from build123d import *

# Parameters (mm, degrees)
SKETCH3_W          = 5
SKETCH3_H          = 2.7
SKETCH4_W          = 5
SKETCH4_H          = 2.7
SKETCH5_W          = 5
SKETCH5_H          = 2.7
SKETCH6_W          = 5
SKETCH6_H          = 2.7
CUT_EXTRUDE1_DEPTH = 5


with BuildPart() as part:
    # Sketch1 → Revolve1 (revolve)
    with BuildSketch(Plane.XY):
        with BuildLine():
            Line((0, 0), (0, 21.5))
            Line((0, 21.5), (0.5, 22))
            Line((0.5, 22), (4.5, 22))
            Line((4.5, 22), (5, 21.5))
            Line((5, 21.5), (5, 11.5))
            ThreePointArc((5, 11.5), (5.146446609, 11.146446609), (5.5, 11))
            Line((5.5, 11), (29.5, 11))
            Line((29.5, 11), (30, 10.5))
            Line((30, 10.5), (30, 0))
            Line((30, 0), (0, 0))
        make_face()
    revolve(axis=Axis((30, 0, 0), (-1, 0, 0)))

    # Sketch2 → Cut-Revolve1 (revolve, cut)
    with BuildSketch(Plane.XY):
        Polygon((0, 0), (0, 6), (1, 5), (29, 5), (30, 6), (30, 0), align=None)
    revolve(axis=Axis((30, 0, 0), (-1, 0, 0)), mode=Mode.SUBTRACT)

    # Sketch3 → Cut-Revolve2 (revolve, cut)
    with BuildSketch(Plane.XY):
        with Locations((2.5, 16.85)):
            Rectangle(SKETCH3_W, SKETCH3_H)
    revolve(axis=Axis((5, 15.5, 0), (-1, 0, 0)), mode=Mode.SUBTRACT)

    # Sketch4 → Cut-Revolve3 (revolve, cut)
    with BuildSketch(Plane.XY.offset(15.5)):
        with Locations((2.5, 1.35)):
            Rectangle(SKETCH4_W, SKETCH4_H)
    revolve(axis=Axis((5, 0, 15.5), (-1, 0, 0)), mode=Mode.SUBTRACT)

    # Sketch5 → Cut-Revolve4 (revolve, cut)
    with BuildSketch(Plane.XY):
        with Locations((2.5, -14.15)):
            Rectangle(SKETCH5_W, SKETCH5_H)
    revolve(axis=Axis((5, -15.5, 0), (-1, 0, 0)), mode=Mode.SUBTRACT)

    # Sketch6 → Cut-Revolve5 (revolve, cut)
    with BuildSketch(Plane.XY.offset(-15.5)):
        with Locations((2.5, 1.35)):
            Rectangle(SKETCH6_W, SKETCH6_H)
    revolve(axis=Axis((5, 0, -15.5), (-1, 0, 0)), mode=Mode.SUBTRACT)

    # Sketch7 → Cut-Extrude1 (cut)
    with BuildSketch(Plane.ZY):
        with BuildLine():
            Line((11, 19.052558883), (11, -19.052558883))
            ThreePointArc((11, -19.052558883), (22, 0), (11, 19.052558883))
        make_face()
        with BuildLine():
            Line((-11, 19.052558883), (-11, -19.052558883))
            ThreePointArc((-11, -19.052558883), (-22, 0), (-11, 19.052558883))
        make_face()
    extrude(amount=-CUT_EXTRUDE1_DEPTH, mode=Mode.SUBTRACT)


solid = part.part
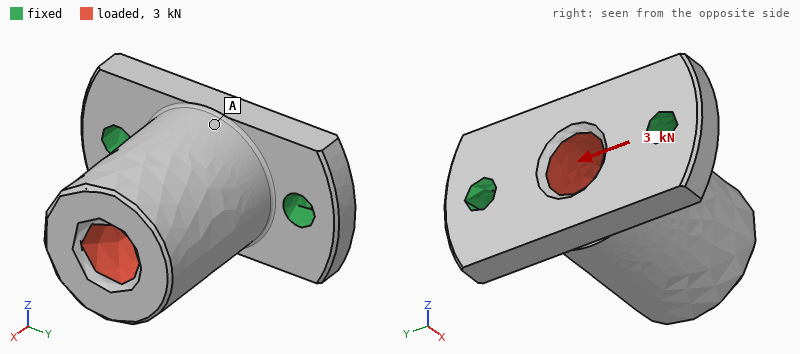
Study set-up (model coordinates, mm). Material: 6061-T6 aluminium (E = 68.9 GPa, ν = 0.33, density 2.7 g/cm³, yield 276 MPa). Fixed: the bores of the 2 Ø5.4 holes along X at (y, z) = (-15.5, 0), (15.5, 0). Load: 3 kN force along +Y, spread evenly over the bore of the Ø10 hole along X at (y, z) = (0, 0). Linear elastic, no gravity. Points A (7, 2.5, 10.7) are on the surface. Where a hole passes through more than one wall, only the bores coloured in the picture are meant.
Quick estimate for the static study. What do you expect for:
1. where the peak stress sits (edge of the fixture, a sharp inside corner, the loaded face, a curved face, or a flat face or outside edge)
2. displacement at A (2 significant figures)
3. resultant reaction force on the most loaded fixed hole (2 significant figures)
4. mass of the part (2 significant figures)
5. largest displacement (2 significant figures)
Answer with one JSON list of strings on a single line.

["a curved face", "5.2 µm", "2.1 kN", "31 g", "30 µm"]
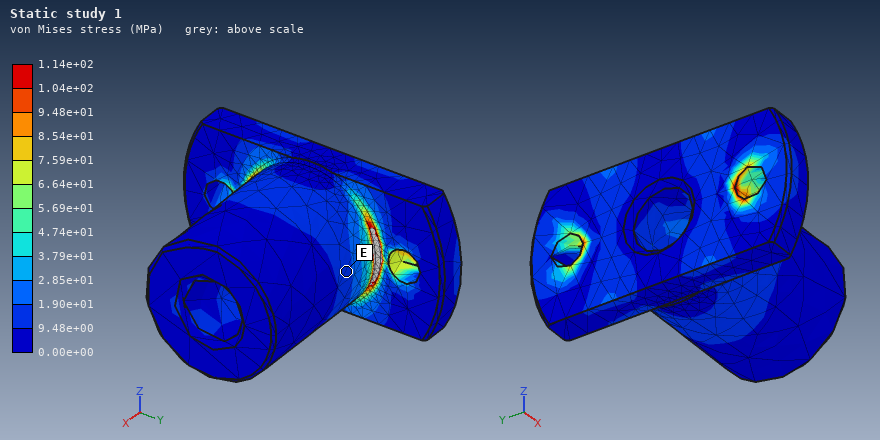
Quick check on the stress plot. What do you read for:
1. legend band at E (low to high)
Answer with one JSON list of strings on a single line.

["9.48e+00 to 1.90e+01 MPa"]
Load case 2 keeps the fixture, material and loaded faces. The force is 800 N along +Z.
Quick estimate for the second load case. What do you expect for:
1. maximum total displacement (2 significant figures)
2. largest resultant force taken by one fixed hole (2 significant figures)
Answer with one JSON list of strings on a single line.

["44 µm", "400 N"]
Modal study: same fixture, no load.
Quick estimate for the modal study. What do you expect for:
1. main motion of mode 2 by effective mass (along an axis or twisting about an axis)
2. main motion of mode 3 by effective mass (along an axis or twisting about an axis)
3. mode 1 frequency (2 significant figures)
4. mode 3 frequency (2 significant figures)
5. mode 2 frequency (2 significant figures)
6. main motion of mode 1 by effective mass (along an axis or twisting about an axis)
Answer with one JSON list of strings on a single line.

["along Y", "along X", "5100 Hz", "17 kHz", "12 kHz", "along Z"]
